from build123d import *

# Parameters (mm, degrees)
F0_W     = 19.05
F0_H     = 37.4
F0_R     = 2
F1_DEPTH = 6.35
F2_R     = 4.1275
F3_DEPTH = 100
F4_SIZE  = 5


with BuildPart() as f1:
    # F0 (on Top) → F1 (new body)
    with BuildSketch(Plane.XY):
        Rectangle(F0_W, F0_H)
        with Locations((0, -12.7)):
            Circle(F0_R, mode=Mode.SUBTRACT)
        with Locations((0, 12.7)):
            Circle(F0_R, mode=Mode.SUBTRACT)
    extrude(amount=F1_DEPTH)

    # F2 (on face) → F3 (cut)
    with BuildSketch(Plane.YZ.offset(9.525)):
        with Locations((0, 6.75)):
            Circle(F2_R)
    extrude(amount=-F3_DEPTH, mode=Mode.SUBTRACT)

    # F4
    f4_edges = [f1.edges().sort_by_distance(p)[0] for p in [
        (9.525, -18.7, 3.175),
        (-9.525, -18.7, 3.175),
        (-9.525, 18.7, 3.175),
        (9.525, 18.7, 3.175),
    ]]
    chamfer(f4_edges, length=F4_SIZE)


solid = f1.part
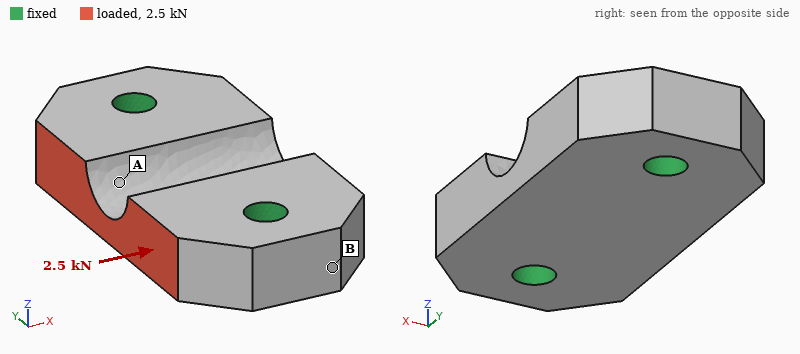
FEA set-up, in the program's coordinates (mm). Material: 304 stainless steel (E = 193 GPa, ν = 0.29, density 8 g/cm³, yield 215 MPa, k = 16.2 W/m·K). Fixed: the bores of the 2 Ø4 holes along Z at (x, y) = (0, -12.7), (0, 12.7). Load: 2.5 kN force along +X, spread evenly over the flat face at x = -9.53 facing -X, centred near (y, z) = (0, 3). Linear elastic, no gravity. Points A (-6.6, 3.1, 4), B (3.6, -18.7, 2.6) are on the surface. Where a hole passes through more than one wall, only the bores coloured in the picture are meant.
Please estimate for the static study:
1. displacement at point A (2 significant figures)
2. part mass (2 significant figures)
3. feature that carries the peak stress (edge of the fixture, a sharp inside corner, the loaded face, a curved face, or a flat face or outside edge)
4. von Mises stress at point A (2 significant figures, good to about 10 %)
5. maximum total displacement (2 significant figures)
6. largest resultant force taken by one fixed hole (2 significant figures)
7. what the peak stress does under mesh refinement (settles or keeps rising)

1.9 µm
29 g
edge of the fixture
14 MPa
2.7 µm
1.3 kN
keeps rising
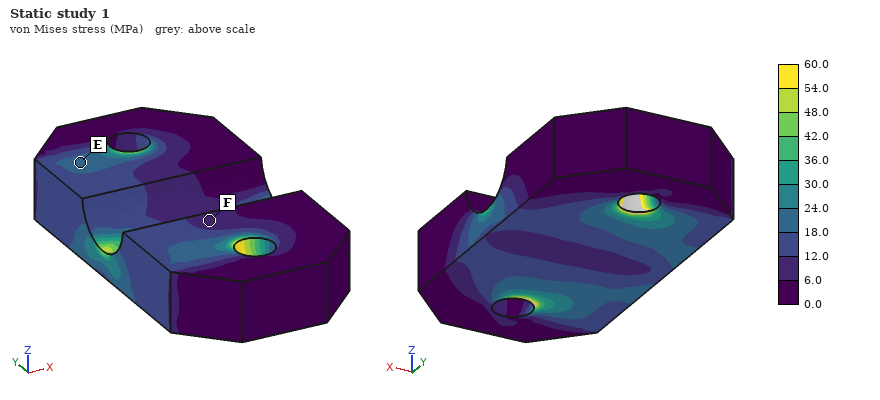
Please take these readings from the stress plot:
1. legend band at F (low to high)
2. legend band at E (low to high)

6.0 to 12.0 MPa
18.0 to 24.0 MPa
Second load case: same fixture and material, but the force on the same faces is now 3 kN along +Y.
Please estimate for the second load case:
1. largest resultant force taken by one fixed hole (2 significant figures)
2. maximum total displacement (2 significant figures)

1.7 kN
3.8 µm
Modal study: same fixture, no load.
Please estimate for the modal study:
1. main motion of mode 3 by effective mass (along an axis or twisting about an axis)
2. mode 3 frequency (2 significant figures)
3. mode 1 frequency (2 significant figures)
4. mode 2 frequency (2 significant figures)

along X
45 kHz
33 kHz
34 kHz
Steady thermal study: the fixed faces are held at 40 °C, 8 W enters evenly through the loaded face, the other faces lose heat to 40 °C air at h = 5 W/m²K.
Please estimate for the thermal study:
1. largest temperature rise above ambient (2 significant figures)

35 K
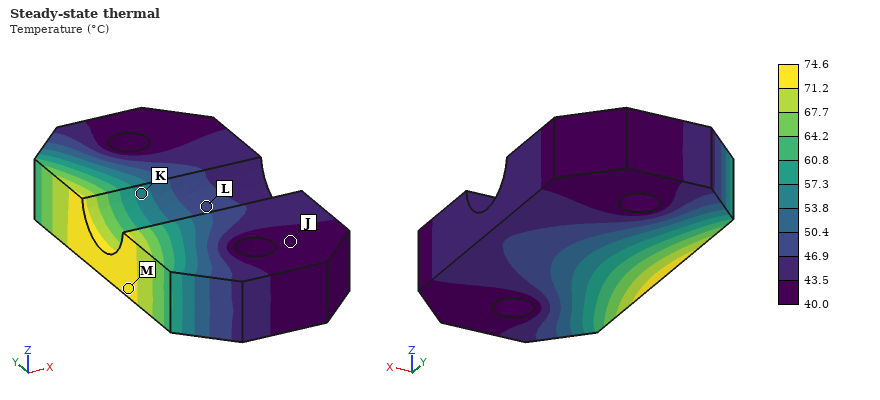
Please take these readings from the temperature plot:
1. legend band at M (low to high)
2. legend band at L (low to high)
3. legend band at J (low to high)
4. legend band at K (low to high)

71.2 to 74.6 °C
46.9 to 50.4 °C
40.0 to 43.5 °C
53.8 to 57.3 °C
